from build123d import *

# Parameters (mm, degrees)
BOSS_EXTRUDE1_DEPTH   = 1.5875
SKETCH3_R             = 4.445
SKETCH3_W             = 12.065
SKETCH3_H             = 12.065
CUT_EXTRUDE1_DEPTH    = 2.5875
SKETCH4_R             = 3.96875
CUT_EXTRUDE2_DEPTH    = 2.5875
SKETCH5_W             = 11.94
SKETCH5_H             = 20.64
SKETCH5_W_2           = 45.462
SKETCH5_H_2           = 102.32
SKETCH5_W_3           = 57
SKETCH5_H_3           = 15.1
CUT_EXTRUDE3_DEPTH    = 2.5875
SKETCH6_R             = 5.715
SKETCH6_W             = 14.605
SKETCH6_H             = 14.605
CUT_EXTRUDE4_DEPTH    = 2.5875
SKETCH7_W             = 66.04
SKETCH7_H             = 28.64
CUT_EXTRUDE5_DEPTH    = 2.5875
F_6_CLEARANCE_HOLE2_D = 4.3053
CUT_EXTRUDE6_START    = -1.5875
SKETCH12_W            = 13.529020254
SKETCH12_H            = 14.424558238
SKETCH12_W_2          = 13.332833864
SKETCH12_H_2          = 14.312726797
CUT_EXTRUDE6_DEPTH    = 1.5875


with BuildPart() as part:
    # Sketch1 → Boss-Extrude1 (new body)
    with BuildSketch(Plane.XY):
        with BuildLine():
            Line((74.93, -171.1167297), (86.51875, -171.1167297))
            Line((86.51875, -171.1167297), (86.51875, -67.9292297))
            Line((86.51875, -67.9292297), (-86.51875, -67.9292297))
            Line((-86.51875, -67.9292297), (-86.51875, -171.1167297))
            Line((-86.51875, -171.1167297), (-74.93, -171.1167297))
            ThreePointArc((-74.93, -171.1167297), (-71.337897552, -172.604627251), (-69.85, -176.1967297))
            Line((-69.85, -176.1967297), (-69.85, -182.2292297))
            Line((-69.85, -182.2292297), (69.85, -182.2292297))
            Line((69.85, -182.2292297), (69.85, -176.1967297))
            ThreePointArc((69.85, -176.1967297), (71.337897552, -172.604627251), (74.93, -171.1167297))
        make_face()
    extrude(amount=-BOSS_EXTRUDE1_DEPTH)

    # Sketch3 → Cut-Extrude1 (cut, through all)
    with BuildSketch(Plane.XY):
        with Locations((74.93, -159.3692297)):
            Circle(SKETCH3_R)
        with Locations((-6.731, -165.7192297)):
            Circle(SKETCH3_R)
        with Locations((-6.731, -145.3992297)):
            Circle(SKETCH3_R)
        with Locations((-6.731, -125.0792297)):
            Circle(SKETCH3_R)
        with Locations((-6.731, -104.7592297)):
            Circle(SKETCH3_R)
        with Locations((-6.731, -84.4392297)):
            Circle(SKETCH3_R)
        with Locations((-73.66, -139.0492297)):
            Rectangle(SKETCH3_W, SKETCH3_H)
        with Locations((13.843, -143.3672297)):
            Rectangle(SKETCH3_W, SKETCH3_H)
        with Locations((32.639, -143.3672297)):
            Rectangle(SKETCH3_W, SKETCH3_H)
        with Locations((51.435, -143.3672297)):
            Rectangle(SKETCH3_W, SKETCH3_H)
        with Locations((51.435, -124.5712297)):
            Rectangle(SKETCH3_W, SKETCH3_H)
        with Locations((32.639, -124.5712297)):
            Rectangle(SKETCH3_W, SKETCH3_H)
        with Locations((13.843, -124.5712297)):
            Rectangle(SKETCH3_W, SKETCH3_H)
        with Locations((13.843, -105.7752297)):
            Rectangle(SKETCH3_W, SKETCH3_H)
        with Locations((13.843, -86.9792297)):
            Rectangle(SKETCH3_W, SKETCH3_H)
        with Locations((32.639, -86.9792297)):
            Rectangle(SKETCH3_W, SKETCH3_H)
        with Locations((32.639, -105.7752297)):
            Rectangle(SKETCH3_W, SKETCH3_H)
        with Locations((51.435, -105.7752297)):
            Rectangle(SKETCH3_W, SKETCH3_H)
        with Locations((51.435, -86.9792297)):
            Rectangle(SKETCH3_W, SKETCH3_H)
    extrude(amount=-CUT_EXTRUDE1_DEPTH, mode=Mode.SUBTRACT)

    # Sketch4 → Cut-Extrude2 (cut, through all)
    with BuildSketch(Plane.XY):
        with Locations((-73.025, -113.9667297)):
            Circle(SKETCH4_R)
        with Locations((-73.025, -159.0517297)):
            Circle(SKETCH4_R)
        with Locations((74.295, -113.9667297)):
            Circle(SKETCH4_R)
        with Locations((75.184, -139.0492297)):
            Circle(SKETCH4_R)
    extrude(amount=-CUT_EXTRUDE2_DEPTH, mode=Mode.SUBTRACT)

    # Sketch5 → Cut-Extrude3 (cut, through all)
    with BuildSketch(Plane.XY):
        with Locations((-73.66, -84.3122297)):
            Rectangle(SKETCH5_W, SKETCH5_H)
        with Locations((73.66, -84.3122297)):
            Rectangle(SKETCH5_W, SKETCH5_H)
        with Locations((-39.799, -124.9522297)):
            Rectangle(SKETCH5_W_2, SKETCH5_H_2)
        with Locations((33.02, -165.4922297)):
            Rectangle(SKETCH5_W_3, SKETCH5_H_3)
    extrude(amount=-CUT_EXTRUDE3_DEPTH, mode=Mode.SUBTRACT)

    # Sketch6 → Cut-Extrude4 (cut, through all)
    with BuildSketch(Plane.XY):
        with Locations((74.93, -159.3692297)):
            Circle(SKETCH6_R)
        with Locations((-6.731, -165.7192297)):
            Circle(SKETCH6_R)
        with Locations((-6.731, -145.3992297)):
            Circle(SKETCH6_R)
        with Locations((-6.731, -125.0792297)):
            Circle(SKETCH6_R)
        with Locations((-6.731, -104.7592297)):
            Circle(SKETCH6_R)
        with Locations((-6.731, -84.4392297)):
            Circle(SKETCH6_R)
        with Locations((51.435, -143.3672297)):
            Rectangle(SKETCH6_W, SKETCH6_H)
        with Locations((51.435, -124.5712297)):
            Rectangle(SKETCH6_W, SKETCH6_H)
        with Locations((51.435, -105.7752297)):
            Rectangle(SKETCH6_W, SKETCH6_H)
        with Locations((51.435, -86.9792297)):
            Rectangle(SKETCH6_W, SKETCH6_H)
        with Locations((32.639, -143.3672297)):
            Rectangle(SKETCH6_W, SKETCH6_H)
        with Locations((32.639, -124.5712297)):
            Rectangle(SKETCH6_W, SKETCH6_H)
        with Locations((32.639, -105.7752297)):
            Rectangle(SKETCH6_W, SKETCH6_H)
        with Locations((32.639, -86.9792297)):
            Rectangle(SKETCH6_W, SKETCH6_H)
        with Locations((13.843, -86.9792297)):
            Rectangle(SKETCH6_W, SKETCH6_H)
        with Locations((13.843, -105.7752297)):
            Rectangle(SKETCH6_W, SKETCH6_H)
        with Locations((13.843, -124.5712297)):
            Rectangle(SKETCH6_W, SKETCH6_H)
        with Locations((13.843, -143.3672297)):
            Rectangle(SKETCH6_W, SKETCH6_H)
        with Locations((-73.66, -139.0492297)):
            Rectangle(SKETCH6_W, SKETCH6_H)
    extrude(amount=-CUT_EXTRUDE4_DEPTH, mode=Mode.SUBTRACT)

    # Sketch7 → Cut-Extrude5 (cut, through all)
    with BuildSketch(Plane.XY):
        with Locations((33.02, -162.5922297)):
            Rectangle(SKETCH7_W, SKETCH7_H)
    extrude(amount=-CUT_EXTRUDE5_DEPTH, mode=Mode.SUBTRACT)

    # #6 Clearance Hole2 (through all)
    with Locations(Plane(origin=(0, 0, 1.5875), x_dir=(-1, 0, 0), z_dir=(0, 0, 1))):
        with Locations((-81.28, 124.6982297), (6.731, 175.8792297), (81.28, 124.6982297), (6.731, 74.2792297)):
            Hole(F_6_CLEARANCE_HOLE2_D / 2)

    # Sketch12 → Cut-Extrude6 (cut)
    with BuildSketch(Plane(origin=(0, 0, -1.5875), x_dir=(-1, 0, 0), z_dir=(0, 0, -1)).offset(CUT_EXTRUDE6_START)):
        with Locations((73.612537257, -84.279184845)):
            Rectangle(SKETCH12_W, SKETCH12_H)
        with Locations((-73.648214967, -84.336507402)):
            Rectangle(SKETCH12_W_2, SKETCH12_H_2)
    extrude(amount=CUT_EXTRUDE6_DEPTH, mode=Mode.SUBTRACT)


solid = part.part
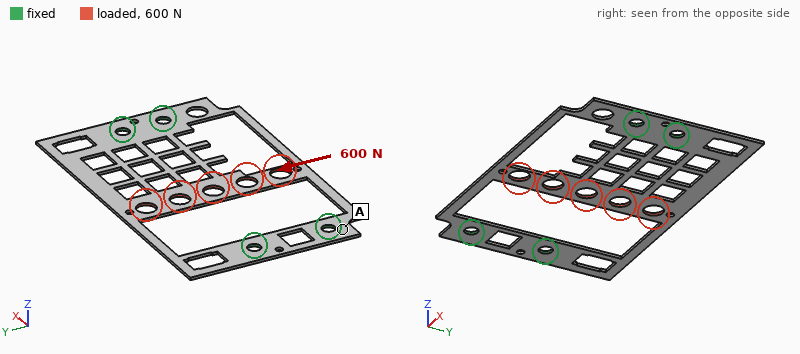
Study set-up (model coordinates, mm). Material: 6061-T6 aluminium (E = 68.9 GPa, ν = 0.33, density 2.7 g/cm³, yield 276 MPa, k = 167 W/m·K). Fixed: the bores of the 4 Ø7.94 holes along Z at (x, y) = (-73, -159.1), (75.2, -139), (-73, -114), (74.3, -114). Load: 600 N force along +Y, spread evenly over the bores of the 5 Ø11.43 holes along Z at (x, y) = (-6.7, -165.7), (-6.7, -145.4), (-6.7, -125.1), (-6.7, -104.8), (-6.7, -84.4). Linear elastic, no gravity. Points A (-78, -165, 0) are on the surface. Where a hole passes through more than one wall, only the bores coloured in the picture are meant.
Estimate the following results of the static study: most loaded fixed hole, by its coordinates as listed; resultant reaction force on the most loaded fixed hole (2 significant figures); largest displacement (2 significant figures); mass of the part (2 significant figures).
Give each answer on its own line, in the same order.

(75.2, -139)
620 N
0.48 mm
38 g
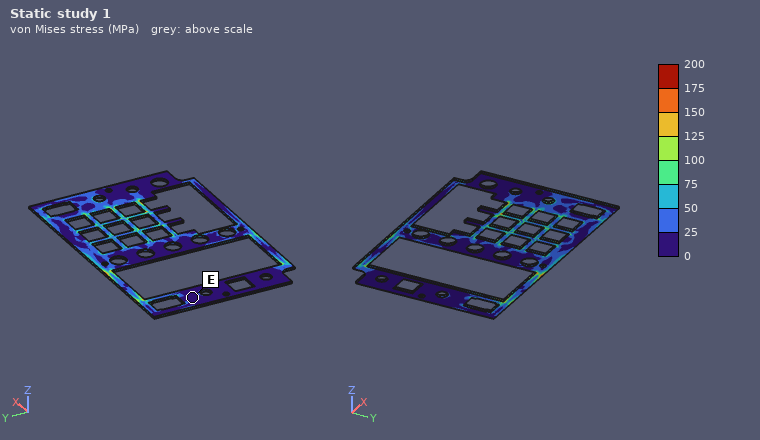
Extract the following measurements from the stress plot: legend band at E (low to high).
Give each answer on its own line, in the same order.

0 to 25 MPa
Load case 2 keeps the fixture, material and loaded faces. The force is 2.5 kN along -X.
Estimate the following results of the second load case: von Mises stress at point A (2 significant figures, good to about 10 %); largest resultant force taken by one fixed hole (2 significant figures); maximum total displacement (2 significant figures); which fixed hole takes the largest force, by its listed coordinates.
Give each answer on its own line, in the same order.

31 MPa
1.5 kN
0.16 mm
(74.3, -114)
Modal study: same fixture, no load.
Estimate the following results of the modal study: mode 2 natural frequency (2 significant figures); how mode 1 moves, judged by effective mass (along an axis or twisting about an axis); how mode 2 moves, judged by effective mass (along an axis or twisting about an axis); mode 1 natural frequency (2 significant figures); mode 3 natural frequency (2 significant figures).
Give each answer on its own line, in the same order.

290 Hz
along Z
twisting about X
220 Hz
510 Hz
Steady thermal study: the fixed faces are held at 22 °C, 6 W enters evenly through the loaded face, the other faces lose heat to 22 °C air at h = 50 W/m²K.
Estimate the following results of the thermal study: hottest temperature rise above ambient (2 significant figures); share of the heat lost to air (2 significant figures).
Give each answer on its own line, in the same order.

17 K
83 %
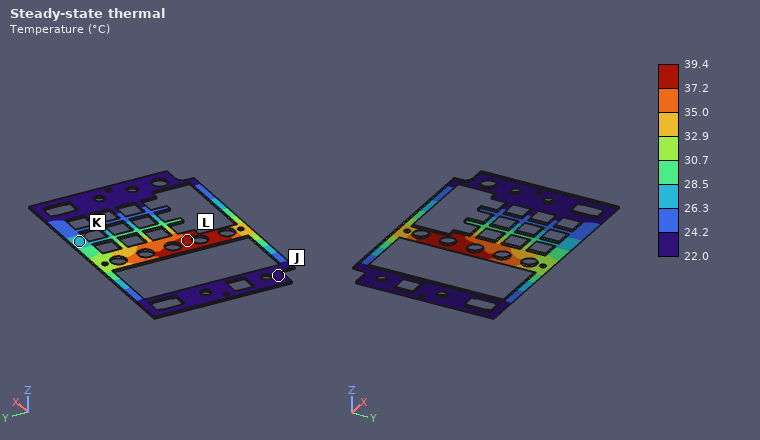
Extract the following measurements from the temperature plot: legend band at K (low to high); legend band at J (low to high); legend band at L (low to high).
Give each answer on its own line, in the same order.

26.3 to 28.5 °C
22.0 to 24.2 °C
37.2 to 39.4 °C
